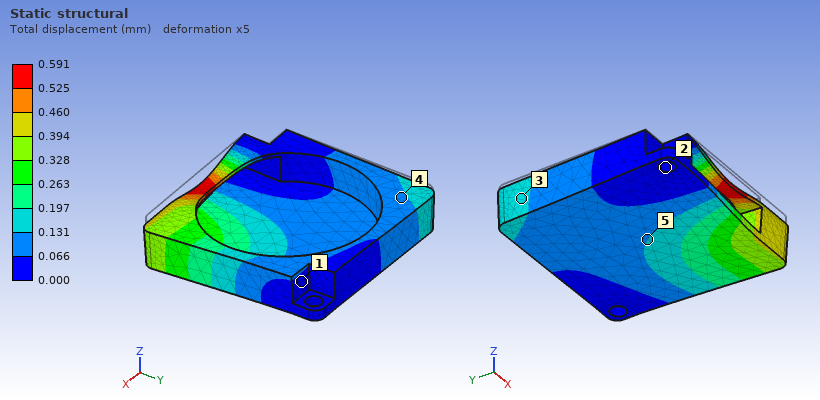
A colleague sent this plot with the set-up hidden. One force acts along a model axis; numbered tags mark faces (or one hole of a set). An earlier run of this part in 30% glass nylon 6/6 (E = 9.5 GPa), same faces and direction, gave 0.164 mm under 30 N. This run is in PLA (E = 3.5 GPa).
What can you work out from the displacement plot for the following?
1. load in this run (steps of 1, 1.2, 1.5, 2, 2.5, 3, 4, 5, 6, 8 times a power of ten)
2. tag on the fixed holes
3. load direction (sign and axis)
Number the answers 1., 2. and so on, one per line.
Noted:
1. 40 N
2. 2
3. -Z
